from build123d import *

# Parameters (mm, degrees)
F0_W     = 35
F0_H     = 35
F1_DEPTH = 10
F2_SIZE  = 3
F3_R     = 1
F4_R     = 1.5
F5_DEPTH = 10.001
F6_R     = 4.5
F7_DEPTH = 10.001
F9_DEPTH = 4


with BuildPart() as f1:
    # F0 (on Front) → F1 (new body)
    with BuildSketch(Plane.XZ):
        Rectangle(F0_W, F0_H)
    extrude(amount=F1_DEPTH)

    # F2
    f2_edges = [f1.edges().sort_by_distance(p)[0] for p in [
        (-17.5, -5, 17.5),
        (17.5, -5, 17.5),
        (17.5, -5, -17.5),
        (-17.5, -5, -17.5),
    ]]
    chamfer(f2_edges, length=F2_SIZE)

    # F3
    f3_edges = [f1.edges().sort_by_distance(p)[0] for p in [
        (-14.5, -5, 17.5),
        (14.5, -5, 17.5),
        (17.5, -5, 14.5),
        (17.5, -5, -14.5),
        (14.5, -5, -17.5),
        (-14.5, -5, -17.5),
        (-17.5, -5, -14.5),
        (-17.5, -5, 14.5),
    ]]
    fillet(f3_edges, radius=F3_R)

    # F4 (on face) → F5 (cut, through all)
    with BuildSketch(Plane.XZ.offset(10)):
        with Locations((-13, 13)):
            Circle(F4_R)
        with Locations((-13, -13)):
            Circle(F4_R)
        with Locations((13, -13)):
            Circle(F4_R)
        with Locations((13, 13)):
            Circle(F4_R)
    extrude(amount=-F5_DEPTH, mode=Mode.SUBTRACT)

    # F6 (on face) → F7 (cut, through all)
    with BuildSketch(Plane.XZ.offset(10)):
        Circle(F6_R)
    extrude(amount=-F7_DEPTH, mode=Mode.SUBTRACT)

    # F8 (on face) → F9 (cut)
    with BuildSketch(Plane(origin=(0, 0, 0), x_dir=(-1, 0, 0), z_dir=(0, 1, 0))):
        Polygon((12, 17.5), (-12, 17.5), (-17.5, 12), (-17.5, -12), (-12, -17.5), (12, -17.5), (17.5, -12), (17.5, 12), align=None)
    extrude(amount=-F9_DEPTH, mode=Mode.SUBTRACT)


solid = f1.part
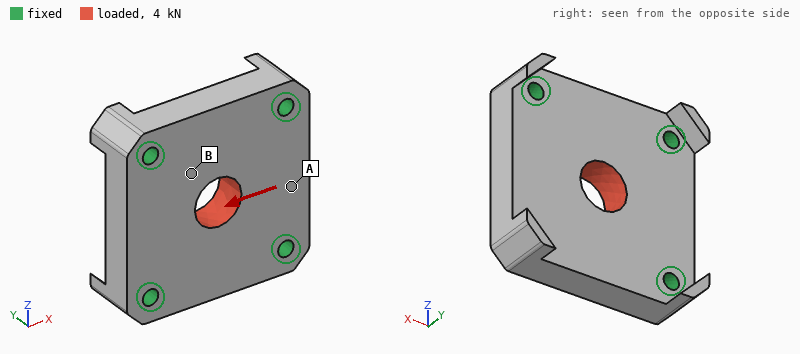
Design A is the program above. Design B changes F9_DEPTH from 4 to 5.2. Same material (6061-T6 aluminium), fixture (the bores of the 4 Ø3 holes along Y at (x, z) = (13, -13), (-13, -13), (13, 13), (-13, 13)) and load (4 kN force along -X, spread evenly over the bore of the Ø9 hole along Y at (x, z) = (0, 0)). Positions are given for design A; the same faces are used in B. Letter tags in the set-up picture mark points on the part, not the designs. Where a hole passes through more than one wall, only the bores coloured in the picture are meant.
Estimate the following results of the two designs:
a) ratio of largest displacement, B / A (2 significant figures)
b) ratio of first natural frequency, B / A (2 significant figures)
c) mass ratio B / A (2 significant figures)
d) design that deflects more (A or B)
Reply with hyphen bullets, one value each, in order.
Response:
- 1.2
- 0.87
- 0.81
- B
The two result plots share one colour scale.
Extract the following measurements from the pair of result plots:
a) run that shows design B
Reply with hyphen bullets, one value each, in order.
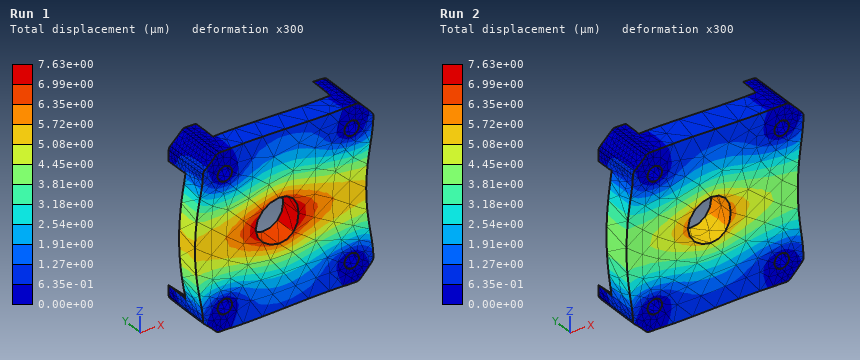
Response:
- Run 1
